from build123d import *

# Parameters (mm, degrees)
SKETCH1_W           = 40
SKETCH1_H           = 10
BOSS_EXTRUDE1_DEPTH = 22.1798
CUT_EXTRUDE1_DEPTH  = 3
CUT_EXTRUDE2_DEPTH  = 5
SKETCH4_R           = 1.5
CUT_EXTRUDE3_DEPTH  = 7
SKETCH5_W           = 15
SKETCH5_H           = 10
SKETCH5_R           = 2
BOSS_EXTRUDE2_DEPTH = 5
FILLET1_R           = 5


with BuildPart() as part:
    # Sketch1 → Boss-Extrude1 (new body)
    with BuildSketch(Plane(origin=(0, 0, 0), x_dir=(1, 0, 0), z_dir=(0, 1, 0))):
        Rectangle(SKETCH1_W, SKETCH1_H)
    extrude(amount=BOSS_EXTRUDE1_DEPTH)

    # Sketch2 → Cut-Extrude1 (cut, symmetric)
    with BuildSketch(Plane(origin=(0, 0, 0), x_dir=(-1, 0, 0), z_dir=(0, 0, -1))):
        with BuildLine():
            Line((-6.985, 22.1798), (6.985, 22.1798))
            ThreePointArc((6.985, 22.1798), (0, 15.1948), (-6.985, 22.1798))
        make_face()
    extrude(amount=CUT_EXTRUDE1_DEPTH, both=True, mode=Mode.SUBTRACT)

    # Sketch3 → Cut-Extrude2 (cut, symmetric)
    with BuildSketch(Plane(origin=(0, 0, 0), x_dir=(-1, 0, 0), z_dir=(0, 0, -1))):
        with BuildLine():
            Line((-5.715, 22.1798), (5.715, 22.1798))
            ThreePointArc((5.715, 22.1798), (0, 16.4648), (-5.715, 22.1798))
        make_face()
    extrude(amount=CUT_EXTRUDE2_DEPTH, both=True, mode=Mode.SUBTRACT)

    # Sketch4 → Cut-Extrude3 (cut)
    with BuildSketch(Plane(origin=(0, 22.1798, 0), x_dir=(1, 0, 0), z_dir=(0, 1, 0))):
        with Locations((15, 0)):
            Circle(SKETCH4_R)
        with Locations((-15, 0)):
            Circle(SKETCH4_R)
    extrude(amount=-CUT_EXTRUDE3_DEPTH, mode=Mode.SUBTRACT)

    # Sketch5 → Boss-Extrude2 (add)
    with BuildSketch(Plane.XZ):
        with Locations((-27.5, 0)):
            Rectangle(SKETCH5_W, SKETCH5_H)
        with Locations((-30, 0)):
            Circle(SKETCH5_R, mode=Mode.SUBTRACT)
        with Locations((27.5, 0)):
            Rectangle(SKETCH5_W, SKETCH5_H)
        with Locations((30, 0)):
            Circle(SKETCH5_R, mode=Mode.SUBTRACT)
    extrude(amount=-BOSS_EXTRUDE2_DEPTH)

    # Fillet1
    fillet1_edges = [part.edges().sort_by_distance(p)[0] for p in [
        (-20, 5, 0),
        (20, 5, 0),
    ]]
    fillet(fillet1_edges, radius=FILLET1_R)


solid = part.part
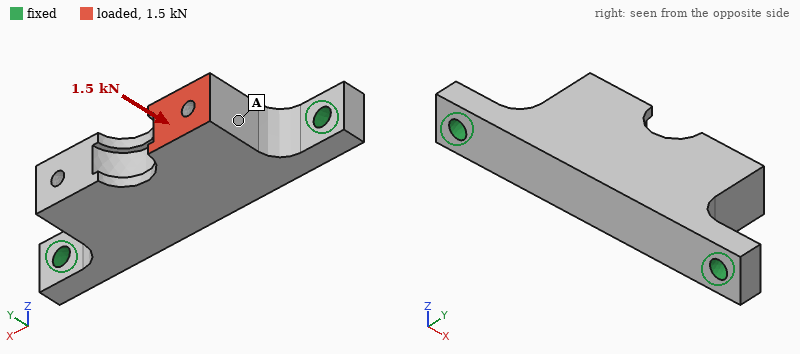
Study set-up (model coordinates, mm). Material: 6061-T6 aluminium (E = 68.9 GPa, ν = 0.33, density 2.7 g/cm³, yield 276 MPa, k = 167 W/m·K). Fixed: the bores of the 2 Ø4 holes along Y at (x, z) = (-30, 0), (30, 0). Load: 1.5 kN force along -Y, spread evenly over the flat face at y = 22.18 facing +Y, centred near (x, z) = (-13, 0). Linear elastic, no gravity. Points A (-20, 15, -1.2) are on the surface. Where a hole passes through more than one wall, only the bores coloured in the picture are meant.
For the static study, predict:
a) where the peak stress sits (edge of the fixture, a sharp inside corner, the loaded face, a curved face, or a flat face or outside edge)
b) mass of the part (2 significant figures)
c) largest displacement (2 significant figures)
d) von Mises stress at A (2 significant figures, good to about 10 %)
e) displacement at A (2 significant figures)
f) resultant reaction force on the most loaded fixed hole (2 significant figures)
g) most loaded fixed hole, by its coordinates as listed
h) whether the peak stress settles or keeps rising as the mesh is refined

edge of the fixture
26 g
25 µm
15 MPa
23 µm
1.3 kN
(-30, 0)
keeps rising
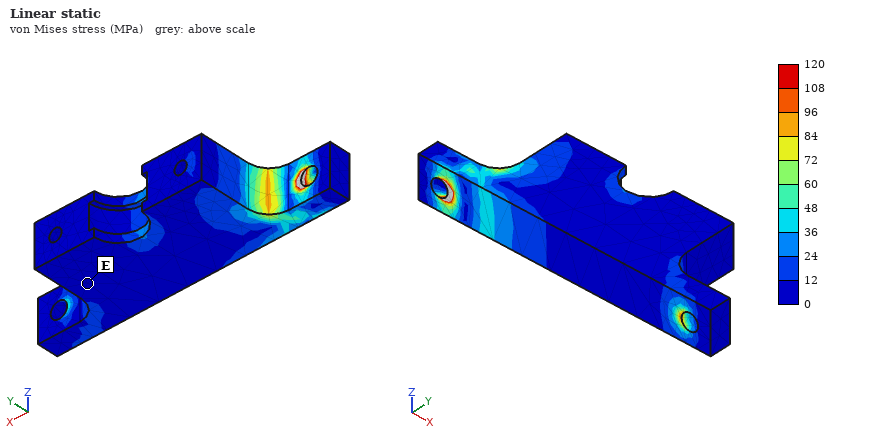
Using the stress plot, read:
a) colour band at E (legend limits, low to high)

0 to 12 MPa
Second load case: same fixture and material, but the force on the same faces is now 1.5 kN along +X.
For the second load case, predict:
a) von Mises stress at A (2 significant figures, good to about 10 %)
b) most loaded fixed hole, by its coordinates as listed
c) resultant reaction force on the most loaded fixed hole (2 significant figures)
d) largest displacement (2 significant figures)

23 MPa
(30, 0)
1.1 kN
26 µm
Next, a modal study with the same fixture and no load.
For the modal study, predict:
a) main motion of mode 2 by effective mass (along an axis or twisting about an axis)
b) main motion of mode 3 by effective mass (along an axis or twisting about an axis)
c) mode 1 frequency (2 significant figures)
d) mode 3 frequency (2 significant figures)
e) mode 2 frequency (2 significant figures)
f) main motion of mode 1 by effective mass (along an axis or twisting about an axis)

along Y
along Z
4200 Hz
12 kHz
9600 Hz
along Z
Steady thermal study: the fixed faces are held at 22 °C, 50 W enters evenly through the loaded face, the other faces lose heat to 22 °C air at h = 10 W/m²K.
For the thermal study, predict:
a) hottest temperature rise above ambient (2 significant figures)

69 K
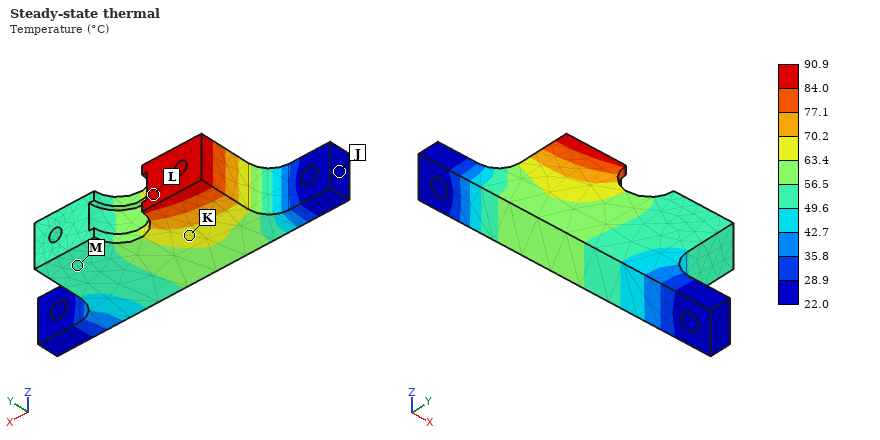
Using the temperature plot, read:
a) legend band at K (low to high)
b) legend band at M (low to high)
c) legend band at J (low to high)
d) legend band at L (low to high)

63.4 to 70.2 °C
49.6 to 56.5 °C
22.0 to 28.9 °C
84.0 to 90.9 °C
